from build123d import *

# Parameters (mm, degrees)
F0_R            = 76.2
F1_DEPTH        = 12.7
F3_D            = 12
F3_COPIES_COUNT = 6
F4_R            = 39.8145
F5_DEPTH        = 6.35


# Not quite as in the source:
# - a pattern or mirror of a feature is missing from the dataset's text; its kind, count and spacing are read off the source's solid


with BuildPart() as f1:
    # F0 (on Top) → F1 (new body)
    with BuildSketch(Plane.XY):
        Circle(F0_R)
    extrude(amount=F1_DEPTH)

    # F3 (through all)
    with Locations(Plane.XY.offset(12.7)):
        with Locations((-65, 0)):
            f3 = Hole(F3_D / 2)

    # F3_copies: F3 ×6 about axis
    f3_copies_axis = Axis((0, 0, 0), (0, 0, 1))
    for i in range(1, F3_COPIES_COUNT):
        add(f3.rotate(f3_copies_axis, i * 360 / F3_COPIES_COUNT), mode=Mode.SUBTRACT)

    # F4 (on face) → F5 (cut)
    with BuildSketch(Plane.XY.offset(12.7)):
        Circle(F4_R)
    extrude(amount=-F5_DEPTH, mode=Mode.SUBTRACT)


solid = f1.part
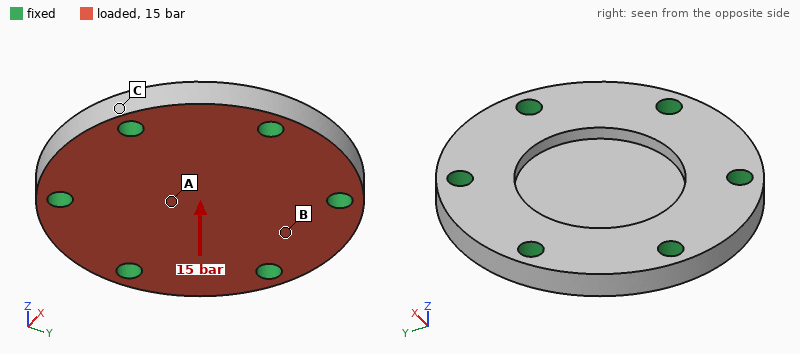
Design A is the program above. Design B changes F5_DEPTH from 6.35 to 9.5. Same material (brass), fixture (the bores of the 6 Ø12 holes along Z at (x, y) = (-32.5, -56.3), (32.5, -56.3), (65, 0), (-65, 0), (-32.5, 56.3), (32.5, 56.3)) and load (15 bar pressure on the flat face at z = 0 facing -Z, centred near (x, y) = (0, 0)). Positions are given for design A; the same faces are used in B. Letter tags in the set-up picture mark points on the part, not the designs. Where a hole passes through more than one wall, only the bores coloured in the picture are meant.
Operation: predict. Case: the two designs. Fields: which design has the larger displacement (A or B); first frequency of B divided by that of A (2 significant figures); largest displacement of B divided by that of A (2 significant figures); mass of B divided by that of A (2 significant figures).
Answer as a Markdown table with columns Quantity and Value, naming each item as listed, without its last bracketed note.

| Quantity | Value |
|---|---|
| which design has the larger displacement | B |
| first frequency of B divided by that of A | 0.72 |
| largest displacement of B divided by that of A | 4.1 |
| mass of B divided by that of A | 0.92 |
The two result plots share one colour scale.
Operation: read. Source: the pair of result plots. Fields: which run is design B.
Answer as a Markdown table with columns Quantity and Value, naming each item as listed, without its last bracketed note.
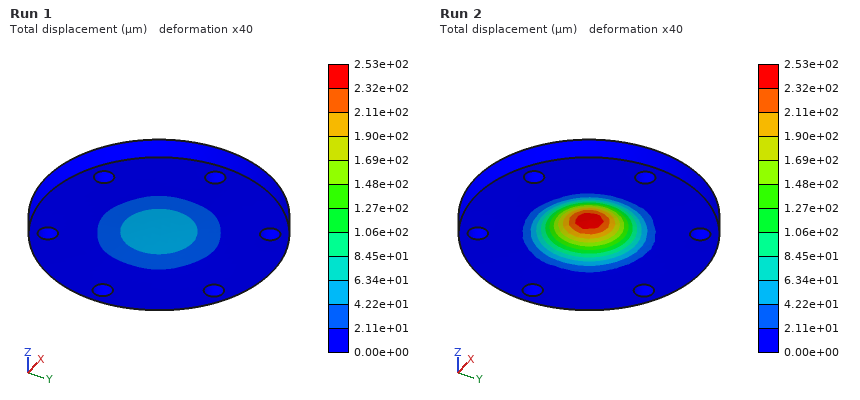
| Quantity | Value |
|---|---|
| which run is design B | Run 2 |
